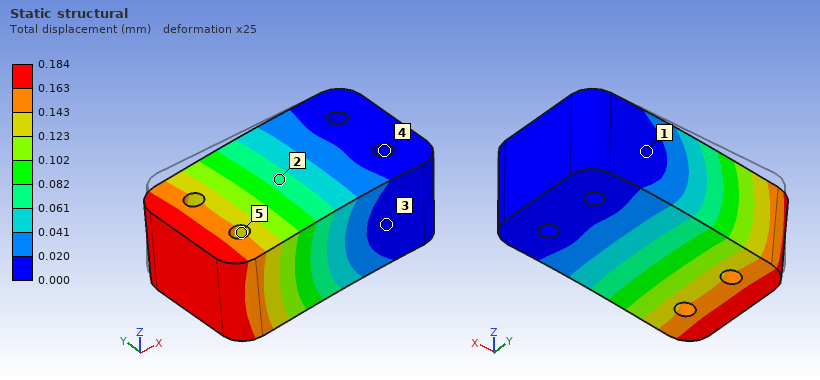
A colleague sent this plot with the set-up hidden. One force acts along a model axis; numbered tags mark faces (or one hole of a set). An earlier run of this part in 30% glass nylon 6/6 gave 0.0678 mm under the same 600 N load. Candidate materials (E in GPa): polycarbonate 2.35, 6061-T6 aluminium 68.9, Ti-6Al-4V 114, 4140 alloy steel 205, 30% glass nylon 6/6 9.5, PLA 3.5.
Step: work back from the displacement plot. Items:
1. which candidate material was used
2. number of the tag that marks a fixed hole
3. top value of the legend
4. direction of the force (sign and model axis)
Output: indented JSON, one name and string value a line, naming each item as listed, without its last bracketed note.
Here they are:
{
  "which candidate material was used": "PLA",
  "number of the tag that marks a fixed hole": "4",
  "top value of the legend": "0.184 mm",
  "direction of the force": "-Z"
}
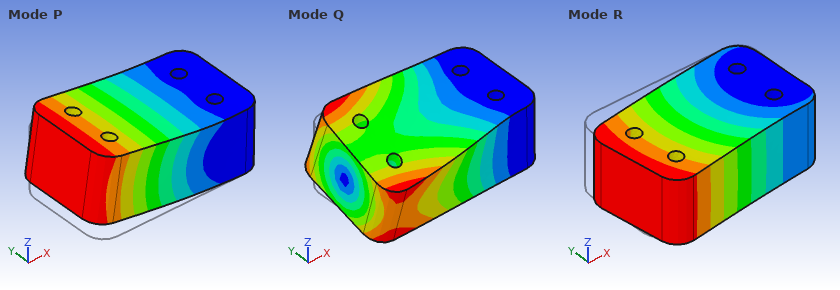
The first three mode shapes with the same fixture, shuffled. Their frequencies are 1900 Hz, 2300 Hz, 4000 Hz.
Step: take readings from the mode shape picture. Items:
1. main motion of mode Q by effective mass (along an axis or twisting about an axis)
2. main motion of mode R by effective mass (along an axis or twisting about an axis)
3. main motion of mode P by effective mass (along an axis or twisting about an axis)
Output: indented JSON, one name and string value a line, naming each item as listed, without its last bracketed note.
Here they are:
{
  "main motion of mode Q by effective mass": "twisting about X",
  "main motion of mode R by effective mass": "along Y",
  "main motion of mode P by effective mass": "along Z"
}
